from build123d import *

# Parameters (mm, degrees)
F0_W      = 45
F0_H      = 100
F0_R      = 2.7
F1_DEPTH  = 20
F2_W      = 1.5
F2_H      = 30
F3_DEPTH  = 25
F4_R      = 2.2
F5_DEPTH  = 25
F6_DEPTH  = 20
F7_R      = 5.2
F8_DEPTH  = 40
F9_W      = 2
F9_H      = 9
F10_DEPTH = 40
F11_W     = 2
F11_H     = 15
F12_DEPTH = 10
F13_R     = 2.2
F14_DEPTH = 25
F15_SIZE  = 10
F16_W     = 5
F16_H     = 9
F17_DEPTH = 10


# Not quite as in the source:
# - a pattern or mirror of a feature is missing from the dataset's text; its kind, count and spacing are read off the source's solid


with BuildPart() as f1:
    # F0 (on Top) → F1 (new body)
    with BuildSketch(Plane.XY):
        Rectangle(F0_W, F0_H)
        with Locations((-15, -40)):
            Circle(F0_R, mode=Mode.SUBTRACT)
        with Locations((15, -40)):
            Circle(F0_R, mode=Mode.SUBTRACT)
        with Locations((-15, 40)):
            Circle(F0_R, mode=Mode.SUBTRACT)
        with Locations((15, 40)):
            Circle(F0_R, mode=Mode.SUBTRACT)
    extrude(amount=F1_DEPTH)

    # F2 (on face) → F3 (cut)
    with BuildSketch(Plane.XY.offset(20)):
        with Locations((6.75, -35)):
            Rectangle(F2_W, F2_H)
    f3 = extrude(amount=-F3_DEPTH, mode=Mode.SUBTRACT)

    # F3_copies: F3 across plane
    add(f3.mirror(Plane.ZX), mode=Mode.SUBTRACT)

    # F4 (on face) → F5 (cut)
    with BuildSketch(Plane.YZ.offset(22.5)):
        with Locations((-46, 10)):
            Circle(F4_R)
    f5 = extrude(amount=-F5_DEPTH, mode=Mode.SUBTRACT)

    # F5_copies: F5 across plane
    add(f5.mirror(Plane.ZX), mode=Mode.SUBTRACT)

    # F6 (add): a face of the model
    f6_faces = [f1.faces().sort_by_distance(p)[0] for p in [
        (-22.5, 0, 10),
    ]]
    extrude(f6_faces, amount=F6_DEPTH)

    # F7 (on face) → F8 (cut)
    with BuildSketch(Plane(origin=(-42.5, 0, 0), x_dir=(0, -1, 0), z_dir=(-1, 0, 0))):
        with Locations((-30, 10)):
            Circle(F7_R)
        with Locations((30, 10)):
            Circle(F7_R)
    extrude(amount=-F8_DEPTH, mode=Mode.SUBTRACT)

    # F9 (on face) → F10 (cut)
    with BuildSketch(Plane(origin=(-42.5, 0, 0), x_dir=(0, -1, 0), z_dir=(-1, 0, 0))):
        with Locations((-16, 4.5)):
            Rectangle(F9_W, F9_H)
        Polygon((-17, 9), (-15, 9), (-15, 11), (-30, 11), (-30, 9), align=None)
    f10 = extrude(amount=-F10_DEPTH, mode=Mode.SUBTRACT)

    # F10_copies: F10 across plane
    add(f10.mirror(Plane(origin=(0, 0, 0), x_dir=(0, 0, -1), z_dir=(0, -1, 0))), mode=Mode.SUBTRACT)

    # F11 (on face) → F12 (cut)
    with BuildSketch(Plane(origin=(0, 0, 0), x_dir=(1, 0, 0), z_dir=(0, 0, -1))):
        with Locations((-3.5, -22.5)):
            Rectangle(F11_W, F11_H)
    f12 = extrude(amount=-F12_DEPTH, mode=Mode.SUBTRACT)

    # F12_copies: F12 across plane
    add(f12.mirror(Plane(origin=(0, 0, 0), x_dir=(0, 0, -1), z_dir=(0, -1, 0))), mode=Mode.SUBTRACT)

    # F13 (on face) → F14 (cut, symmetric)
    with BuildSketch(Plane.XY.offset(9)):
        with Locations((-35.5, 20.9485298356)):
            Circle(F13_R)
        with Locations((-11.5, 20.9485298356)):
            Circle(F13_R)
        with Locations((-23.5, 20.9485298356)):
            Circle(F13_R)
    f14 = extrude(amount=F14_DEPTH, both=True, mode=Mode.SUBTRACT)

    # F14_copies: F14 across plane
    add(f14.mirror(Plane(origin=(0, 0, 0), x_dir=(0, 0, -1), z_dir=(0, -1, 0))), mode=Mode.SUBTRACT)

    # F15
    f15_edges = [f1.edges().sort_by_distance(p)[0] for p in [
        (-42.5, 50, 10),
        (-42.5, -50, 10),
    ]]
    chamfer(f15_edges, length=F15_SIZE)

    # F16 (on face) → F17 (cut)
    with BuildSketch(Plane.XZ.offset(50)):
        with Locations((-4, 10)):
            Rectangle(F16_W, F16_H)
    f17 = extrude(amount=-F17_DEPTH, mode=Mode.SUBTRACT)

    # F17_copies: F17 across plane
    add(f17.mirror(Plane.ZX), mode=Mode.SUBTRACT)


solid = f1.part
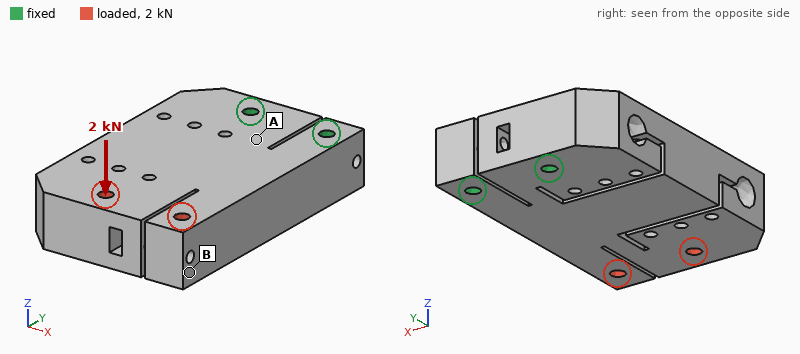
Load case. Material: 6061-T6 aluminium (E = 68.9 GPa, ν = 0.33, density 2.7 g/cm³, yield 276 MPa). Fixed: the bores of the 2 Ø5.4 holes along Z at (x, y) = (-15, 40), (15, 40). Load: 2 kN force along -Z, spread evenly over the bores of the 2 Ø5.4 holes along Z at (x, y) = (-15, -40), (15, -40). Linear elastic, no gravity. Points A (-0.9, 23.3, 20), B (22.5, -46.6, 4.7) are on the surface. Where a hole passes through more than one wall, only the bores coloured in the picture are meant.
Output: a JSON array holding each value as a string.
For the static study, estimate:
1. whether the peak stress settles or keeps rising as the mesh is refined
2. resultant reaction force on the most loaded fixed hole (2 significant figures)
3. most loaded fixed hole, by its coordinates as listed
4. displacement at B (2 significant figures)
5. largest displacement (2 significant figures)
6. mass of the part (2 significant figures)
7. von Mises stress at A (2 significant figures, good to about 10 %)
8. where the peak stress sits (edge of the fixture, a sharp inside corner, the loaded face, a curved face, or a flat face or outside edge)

["keeps rising", "1.5 kN", "(15, 40)", "0.32 mm", "0.39 mm", "300 g", "44 MPa", "edge of the fixture"]
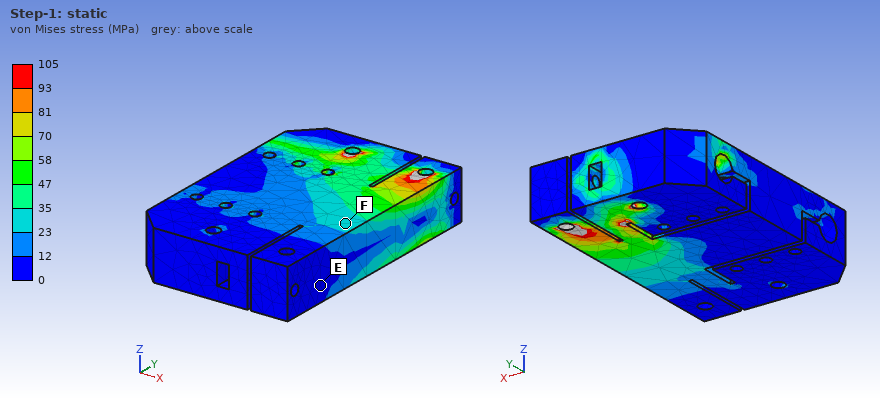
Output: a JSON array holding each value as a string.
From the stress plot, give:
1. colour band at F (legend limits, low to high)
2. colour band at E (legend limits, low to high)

["23 to 35 MPa", "0 to 12 MPa"]
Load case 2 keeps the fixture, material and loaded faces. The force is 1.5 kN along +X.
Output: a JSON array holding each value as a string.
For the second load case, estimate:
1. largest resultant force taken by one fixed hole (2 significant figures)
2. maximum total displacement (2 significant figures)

["3.4 kN", "79 µm"]
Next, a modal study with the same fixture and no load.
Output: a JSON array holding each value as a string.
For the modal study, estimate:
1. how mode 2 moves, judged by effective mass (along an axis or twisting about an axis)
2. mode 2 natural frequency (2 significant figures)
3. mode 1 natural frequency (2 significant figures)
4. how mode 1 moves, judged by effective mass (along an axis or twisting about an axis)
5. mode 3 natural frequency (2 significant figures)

["along X", "2800 Hz", "1200 Hz", "along Z", "3500 Hz"]
